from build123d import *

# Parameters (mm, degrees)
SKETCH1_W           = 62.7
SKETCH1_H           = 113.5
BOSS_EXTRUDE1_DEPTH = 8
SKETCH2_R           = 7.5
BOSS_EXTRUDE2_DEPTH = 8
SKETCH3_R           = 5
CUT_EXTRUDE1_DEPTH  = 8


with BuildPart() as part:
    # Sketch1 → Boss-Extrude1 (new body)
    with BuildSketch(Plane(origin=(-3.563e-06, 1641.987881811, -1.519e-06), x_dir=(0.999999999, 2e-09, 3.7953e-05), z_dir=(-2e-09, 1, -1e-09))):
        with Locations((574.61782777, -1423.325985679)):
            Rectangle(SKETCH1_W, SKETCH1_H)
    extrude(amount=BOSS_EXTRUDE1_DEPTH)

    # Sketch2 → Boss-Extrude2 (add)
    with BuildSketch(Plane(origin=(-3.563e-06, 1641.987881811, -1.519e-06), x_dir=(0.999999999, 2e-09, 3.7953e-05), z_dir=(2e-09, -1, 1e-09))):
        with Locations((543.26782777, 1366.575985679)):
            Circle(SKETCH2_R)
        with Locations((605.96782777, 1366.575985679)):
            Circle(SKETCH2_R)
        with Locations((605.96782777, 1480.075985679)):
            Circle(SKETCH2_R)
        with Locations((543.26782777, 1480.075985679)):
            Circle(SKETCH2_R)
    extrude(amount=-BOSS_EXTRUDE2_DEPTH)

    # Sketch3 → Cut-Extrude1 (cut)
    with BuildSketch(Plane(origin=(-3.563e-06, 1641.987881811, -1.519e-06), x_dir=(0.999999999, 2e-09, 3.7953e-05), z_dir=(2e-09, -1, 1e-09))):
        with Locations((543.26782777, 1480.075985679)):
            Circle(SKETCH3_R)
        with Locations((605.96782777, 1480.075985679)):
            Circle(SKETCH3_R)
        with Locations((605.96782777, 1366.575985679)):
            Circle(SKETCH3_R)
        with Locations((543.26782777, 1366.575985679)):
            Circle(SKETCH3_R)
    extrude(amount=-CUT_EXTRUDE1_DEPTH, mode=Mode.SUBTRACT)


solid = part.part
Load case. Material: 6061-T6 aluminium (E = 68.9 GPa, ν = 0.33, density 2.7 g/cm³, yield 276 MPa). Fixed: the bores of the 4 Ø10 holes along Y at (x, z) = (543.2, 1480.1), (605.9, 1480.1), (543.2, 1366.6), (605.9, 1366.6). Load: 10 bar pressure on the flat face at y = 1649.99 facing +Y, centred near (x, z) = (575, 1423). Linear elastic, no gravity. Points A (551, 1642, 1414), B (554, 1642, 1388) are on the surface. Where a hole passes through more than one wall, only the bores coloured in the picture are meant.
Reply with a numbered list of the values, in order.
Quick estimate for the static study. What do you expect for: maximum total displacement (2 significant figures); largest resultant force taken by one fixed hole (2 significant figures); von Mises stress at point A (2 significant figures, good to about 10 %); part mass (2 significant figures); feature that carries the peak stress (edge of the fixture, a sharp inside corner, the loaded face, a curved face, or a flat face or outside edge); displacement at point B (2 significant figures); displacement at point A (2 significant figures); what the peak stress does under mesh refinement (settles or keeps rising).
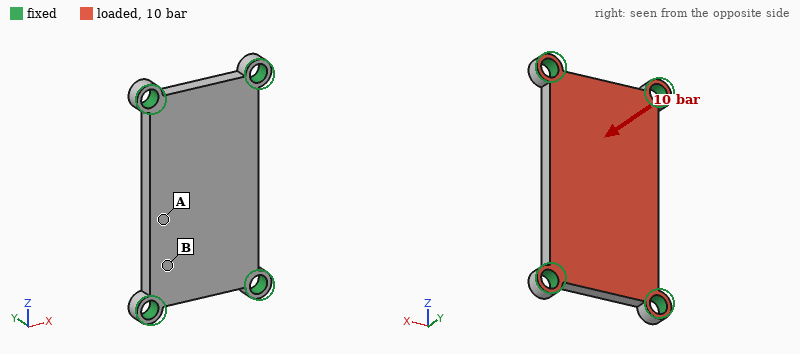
1. 0.21 mm
2. 1.8 kN
3. 57 MPa
4. 160 g
5. edge of the fixture
6. 0.091 mm
7. 0.19 mm
8. keeps rising
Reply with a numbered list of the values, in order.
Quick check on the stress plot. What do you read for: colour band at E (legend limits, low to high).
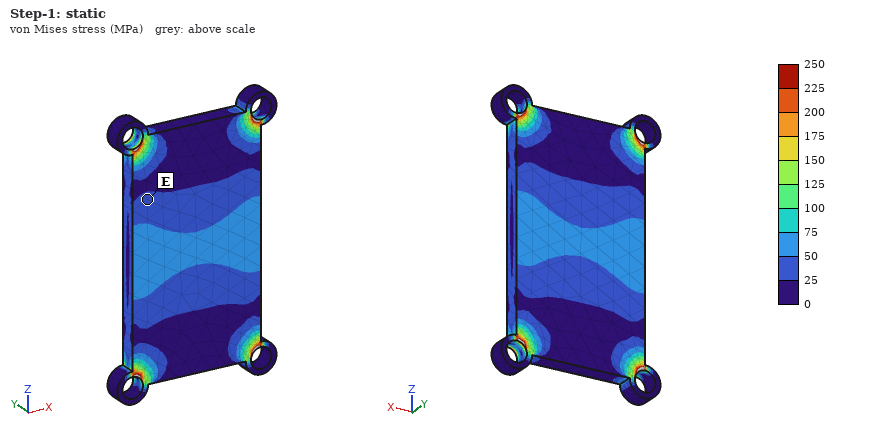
1. 25 to 50 MPa
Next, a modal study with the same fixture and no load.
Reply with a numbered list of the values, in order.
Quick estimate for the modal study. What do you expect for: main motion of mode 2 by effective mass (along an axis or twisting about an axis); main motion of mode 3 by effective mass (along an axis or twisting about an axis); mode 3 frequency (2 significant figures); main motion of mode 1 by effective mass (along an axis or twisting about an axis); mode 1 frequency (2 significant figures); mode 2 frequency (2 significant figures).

1. twisting about Z
2. twisting about X
3. 7300 Hz
4. along Y
5. 2700 Hz
6. 4900 Hz
